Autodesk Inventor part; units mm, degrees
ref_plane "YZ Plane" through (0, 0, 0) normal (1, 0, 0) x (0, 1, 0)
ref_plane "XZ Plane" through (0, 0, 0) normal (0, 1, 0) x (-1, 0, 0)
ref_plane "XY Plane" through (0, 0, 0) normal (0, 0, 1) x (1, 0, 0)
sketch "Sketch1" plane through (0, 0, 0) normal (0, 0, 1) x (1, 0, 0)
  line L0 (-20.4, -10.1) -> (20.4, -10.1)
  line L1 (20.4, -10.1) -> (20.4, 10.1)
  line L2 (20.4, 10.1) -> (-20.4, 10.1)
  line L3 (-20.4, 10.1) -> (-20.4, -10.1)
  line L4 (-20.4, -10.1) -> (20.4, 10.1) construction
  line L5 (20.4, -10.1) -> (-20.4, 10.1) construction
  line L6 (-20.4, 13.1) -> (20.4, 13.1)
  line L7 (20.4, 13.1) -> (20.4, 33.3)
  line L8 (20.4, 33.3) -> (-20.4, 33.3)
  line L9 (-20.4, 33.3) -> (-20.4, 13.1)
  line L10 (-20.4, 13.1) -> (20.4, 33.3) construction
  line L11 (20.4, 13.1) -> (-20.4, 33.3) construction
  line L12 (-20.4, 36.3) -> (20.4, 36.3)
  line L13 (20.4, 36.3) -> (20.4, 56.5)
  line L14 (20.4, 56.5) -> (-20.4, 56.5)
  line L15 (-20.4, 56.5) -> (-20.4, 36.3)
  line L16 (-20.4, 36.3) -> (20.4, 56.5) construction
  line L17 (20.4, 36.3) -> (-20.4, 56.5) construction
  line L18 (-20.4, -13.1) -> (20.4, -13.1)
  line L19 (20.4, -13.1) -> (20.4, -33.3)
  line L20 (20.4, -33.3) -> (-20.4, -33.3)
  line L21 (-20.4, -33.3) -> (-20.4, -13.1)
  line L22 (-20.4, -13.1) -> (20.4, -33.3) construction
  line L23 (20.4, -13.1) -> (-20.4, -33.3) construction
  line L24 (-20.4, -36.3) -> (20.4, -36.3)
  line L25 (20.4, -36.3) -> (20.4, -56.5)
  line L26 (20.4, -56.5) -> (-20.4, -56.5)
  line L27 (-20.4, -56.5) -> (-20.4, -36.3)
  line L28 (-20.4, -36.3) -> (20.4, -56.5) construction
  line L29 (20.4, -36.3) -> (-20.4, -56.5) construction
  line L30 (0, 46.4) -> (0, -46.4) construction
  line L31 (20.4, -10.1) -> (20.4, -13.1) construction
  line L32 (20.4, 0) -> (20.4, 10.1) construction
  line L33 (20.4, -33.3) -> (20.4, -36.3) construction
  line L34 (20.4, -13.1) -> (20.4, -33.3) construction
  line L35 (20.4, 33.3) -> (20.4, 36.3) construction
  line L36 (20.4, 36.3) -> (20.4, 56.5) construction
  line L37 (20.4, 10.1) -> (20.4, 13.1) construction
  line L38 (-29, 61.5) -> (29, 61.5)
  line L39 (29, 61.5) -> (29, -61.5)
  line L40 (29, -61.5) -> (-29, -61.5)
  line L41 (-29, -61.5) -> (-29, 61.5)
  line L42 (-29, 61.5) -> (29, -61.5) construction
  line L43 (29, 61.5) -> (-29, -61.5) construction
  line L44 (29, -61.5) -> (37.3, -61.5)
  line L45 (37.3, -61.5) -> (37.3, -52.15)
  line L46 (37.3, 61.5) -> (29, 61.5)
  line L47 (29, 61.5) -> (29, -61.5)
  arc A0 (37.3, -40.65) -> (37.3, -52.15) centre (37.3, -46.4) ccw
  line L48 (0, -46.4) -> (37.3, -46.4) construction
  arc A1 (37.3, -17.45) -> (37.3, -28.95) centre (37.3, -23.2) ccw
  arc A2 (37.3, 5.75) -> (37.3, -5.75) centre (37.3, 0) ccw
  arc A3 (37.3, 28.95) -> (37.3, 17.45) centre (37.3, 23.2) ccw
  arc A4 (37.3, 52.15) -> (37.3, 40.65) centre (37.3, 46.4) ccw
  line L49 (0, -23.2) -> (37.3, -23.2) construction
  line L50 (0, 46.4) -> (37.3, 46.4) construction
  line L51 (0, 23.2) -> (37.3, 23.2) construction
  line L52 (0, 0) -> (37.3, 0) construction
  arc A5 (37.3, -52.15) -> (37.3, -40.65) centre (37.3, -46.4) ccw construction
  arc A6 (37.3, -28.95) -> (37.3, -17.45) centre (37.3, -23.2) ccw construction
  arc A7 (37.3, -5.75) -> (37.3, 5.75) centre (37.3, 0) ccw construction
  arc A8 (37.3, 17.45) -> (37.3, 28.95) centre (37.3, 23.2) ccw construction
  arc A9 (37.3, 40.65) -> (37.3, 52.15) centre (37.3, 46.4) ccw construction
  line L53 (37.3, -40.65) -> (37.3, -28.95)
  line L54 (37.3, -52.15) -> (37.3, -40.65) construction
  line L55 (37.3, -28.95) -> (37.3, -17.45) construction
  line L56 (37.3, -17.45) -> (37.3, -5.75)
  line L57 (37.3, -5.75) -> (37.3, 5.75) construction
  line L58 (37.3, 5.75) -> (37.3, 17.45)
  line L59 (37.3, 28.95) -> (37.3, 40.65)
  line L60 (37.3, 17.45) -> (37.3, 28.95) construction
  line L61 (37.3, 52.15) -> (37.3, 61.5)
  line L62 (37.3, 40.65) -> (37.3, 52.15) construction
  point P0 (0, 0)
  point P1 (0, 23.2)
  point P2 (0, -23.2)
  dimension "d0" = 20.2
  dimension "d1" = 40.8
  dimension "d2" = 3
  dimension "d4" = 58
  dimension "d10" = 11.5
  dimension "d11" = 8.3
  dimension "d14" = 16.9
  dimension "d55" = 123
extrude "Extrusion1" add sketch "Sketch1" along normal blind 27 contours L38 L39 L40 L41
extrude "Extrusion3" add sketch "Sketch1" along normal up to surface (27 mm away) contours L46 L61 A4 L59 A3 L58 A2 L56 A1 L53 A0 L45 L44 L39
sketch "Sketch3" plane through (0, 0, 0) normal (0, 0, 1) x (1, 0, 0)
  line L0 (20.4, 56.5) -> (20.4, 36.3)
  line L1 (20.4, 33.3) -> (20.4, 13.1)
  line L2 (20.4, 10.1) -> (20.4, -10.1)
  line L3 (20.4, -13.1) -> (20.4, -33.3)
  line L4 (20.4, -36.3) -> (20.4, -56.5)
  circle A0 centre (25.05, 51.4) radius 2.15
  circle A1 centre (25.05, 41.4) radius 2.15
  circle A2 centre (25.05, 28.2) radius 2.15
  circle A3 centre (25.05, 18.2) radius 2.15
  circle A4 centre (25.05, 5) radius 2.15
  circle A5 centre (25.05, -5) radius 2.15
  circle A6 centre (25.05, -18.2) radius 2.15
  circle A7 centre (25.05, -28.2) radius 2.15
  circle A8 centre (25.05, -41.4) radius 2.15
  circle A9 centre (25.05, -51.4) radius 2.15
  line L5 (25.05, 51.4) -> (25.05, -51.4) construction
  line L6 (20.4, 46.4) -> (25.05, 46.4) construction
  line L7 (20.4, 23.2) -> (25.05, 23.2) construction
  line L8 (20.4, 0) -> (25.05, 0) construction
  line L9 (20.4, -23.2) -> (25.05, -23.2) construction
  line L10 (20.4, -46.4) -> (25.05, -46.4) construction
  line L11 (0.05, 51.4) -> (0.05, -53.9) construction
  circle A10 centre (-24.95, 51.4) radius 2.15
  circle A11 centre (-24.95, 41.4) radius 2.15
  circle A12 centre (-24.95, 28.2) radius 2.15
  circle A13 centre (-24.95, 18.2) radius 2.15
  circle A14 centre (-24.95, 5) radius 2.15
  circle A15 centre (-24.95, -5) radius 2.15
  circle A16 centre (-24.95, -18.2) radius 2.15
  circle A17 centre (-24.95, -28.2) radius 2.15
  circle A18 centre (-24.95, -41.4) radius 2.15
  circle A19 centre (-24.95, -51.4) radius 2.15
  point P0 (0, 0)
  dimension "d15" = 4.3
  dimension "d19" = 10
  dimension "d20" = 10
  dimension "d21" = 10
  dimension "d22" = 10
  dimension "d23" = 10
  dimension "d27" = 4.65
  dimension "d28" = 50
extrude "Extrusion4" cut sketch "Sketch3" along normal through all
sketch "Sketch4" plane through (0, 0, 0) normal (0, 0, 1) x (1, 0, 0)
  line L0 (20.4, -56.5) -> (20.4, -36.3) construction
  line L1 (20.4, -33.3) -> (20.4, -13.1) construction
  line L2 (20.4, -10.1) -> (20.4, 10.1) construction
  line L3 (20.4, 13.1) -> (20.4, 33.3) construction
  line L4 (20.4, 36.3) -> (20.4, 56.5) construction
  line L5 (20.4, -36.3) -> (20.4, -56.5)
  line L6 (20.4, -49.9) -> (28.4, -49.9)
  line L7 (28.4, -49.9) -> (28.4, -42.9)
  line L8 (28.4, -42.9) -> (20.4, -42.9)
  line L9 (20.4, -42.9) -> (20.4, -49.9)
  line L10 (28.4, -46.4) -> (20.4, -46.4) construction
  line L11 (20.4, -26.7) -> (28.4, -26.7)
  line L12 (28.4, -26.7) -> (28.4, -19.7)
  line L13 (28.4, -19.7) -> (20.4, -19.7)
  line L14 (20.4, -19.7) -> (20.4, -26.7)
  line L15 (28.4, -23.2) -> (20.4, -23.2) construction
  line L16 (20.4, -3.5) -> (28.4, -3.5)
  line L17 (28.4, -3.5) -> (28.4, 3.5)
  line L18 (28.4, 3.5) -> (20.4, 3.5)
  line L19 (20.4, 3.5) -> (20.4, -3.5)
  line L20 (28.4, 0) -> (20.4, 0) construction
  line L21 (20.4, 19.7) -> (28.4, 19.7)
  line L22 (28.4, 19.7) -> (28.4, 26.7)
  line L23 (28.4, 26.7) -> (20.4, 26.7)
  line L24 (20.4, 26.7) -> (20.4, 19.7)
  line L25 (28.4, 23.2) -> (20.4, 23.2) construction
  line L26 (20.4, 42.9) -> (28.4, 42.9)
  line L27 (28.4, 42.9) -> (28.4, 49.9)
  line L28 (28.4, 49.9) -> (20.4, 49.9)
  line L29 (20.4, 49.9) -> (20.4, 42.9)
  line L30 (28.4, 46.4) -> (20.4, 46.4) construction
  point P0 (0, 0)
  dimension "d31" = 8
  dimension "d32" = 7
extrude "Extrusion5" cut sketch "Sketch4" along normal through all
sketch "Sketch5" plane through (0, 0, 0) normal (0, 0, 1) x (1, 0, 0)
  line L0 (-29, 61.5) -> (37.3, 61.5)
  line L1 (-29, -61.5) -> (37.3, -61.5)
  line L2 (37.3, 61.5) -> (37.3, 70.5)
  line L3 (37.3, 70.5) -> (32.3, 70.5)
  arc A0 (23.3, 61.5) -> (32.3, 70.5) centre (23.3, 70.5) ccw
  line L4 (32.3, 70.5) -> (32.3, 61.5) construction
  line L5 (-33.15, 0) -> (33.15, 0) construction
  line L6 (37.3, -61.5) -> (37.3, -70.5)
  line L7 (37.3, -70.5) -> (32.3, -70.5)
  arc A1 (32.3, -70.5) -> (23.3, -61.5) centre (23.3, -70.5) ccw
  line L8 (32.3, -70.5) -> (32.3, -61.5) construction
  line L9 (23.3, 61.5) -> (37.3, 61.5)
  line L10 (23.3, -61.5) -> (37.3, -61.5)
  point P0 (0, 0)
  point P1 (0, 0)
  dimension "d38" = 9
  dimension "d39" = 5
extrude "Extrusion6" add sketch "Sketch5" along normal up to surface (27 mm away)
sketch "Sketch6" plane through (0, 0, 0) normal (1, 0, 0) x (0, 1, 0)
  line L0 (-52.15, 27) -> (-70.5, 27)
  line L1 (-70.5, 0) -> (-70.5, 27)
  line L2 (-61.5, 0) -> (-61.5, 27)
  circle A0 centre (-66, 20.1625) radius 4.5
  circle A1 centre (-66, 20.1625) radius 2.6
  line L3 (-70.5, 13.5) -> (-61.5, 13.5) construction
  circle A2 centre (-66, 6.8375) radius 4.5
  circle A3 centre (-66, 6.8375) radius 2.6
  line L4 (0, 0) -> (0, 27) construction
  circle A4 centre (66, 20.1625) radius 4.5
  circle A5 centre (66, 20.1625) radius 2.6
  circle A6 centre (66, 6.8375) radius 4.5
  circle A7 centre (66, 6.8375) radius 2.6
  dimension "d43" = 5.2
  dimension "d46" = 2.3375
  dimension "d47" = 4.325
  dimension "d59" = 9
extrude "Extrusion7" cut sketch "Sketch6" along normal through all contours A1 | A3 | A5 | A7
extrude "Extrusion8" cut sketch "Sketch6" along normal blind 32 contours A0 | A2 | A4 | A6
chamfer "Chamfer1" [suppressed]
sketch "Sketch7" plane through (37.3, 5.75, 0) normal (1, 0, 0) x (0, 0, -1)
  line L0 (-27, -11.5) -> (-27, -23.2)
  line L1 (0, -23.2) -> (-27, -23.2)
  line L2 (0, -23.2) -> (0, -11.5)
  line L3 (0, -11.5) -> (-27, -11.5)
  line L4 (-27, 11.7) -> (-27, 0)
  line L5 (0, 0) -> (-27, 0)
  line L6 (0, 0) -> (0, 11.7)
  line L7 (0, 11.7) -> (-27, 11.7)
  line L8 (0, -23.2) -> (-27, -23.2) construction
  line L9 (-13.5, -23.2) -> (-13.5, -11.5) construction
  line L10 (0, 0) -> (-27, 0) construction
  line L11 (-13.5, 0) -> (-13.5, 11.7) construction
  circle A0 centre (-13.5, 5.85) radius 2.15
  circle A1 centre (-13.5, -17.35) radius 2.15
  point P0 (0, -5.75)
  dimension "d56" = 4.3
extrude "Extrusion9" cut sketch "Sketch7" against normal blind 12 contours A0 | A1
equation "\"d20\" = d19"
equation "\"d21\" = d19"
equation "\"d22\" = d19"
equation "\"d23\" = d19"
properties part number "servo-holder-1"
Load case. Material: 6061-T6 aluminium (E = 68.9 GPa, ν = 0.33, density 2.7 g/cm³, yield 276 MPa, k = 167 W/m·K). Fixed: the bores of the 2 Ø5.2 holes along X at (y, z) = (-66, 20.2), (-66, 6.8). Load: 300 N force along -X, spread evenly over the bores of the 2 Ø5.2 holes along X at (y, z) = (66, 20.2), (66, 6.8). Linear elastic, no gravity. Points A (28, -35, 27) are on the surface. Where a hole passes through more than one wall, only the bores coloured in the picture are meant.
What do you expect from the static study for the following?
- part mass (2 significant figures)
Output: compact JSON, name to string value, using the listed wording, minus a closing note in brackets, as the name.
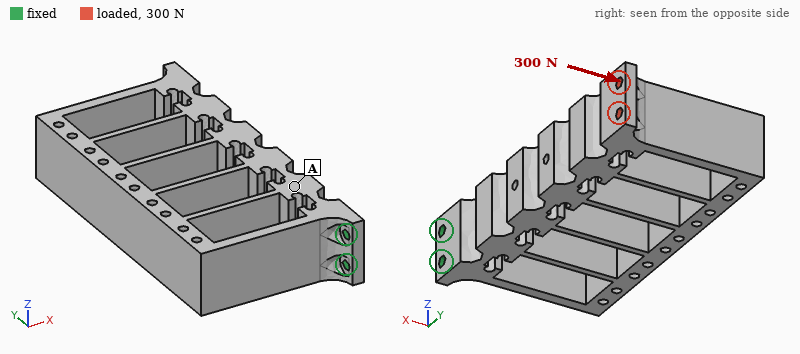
{"part mass": "240 g"}
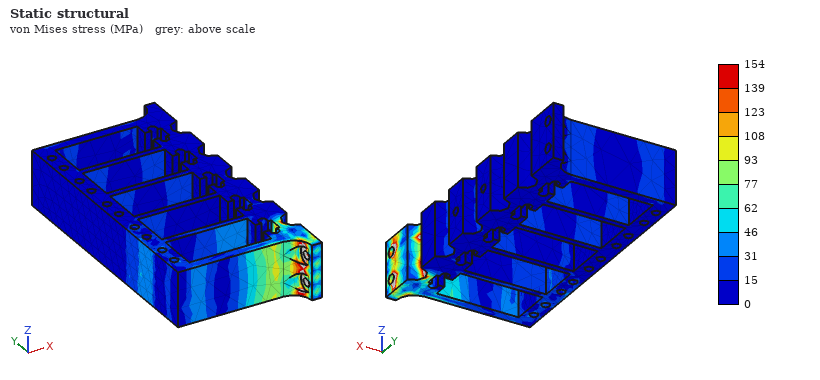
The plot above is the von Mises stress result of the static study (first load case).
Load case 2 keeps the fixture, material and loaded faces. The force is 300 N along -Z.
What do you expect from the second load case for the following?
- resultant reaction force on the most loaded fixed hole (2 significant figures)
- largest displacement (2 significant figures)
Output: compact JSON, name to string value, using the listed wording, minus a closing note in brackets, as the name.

{"resultant reaction force on the most loaded fixed hole": "2.3 kN", "largest displacement": "0.41 mm"}
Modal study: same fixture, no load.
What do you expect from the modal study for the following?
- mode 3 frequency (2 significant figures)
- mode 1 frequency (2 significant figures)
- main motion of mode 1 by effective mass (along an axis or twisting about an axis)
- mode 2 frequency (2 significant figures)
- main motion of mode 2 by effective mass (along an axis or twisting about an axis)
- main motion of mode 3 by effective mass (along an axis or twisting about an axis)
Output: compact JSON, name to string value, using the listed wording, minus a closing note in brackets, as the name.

{"mode 3 frequency": "1000 Hz", "mode 1 frequency": "220 Hz", "main motion of mode 1 by effective mass": "along X", "mode 2 frequency": "470 Hz", "main motion of mode 2 by effective mass": "along Z", "main motion of mode 3 by effective mass": "twisting about Y"}
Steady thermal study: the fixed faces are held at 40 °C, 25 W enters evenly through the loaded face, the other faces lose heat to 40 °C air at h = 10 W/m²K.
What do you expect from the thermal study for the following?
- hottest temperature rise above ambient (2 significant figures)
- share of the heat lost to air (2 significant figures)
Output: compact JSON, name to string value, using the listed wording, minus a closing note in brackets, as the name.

{"hottest temperature rise above ambient": "64 K", "share of the heat lost to air": "44 %"}
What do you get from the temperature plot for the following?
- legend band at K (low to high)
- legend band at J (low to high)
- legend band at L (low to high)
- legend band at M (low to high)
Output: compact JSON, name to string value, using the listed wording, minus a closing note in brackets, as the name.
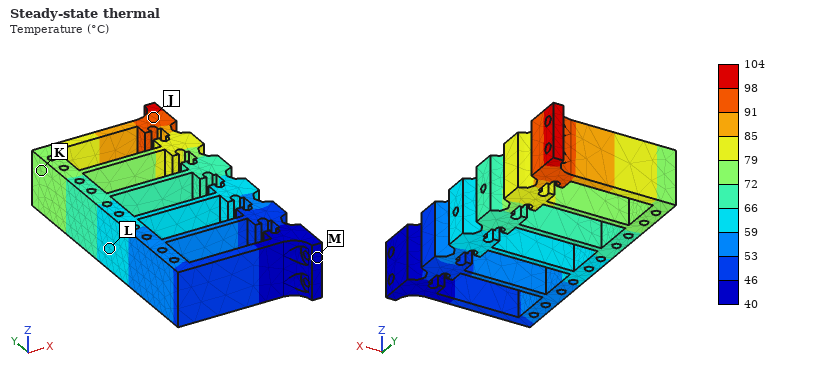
{"legend band at K": "72 to 79 °C", "legend band at J": "91 to 98 °C", "legend band at L": "59 to 66 °C", "legend band at M": "40 to 46 °C"}
